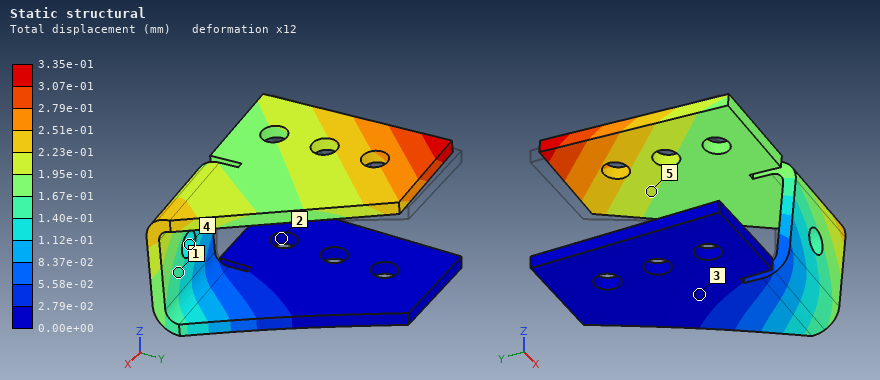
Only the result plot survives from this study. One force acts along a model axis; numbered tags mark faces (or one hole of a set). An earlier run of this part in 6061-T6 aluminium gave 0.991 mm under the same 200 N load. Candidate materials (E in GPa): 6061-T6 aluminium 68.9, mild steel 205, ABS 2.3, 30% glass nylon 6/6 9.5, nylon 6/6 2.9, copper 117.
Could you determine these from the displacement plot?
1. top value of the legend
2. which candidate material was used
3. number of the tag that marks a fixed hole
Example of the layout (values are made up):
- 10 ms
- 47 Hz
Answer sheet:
- 3.35e-01 mm
- mild steel
- 2
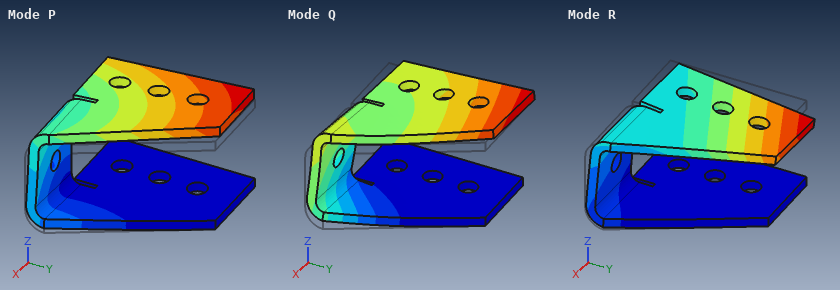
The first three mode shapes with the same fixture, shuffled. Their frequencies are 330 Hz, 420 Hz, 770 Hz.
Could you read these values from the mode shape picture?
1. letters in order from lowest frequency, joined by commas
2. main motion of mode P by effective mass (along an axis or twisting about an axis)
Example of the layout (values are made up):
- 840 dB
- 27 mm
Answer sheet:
- R, P, Q
- along X
